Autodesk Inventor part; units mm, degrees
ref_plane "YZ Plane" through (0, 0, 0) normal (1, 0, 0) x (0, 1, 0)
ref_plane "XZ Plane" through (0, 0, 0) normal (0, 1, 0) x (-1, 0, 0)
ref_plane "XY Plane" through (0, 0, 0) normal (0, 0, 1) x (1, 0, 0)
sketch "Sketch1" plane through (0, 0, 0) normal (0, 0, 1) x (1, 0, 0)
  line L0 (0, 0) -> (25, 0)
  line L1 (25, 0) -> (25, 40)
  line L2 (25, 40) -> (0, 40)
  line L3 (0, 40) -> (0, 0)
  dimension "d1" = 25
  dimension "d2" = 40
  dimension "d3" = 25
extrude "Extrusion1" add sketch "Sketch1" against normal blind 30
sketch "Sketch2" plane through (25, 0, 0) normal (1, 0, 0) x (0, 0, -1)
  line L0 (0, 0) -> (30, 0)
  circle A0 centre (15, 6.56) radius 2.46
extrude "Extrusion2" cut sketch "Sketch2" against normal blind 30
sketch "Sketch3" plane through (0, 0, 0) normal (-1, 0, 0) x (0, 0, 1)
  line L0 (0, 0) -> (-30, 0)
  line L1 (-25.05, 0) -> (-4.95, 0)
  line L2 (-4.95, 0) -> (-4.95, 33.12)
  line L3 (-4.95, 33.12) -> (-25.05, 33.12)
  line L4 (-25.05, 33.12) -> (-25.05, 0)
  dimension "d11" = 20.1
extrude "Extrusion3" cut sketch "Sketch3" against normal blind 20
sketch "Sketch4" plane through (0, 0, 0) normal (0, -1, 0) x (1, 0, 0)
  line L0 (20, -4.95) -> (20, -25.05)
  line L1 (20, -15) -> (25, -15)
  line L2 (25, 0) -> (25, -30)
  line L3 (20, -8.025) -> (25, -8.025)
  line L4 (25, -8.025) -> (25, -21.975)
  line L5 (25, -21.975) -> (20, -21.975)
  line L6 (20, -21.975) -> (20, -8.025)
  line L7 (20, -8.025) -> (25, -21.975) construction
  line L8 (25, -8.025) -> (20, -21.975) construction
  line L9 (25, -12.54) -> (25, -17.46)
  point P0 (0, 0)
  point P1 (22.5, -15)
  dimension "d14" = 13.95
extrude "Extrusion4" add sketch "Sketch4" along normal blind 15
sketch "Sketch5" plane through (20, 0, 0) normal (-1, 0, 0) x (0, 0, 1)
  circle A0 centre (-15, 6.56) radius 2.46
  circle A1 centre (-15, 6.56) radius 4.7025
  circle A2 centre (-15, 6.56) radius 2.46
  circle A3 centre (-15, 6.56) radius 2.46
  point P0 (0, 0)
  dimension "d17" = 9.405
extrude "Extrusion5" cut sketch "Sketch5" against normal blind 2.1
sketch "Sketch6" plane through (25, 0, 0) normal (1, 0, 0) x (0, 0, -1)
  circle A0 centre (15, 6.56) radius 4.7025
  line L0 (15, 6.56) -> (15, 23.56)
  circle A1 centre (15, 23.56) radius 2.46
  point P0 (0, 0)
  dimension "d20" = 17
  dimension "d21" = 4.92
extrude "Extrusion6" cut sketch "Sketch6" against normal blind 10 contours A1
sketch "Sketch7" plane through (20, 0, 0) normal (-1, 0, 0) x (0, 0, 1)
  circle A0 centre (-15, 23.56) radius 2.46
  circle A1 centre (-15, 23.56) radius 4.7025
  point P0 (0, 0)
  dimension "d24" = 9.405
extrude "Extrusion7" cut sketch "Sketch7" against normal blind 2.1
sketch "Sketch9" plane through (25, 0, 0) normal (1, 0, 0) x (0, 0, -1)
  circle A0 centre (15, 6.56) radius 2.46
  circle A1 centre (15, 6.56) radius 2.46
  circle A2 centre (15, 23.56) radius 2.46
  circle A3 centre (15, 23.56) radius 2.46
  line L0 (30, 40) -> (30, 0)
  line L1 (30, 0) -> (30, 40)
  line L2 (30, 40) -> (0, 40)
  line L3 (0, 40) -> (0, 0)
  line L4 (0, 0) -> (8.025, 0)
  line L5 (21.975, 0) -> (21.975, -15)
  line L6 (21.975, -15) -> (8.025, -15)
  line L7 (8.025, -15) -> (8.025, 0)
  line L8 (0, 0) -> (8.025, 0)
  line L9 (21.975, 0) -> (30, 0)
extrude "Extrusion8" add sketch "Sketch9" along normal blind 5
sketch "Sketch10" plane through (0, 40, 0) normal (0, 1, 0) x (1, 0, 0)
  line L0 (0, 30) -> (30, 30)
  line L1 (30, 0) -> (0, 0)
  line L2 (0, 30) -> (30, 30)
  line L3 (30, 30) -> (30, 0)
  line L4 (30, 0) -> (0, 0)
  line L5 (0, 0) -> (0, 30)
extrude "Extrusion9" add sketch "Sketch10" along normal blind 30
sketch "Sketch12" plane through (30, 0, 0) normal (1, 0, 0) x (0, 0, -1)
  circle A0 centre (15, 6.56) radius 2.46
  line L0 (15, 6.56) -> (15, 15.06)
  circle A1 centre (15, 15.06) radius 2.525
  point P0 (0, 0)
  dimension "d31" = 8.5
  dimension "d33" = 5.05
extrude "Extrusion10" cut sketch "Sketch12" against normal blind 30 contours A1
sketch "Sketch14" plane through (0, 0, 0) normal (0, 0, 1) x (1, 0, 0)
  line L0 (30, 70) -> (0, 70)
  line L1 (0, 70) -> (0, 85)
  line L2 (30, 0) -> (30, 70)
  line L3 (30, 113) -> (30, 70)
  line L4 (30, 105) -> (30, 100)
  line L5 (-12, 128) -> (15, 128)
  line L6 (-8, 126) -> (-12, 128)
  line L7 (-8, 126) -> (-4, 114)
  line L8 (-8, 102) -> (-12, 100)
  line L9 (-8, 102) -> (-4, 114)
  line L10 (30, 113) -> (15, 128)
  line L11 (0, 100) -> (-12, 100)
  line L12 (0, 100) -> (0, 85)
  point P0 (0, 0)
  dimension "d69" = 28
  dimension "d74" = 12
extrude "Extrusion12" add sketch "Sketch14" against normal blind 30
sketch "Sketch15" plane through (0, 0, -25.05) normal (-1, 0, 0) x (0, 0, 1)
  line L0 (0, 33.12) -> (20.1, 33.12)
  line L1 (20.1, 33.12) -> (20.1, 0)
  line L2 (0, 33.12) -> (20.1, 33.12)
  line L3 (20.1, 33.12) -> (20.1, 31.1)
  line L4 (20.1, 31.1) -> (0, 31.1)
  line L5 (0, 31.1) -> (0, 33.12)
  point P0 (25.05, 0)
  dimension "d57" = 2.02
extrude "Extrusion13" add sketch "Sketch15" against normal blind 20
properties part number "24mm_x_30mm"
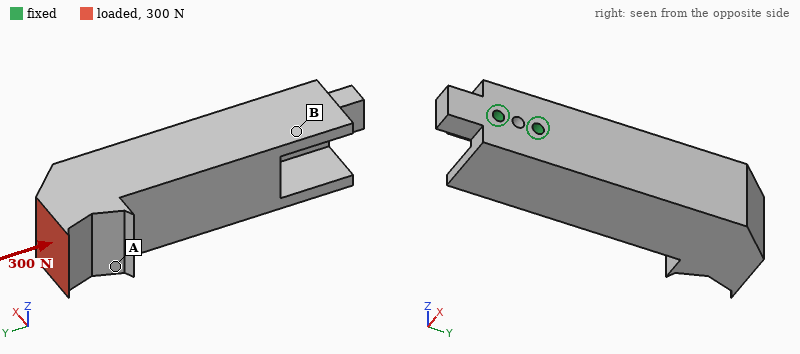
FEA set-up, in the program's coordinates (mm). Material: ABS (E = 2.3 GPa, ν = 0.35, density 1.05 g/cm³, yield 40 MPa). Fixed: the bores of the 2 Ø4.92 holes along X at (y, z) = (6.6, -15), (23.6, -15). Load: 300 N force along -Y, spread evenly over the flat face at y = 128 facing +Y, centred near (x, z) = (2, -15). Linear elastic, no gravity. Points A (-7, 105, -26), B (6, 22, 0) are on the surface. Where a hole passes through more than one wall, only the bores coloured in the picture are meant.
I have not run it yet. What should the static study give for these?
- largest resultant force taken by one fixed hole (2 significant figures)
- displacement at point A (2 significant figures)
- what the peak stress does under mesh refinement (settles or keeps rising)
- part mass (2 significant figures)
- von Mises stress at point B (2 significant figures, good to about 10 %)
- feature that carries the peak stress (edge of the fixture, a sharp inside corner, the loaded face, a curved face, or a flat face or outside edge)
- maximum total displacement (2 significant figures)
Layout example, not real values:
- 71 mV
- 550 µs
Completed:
- 340 N
- 0.51 mm
- keeps rising
- 110 g
- 1.9 MPa
- edge of the fixture
- 0.70 mm
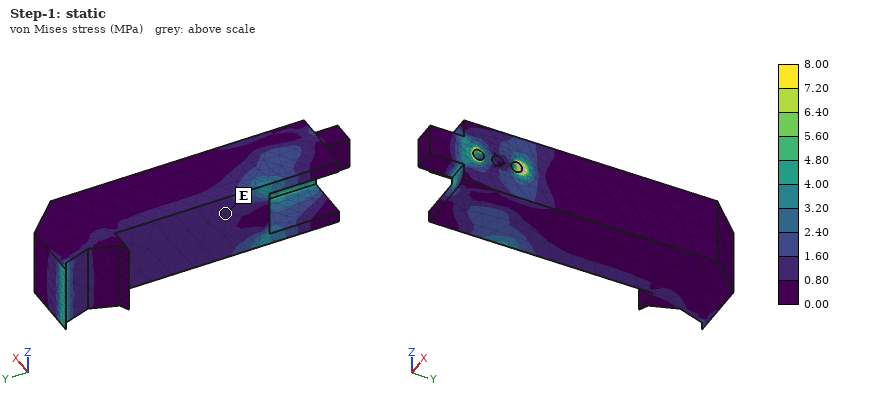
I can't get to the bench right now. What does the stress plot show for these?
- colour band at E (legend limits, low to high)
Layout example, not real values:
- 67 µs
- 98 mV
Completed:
- 0.80 to 1.60 MPa
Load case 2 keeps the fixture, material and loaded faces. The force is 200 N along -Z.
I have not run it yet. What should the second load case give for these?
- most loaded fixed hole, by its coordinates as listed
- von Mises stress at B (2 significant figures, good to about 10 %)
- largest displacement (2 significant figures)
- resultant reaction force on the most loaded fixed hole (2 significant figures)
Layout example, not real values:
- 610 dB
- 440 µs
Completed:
- (23.6, -15)
- 3.4 MPa
- 1.6 mm
- 1.1 kN
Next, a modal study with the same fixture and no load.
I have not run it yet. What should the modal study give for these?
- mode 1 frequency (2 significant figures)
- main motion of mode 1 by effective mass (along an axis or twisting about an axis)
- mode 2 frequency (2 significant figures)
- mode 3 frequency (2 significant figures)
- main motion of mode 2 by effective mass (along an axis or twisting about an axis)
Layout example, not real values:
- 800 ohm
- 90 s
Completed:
- 280 Hz
- along X
- 330 Hz
- 900 Hz
- along Z
